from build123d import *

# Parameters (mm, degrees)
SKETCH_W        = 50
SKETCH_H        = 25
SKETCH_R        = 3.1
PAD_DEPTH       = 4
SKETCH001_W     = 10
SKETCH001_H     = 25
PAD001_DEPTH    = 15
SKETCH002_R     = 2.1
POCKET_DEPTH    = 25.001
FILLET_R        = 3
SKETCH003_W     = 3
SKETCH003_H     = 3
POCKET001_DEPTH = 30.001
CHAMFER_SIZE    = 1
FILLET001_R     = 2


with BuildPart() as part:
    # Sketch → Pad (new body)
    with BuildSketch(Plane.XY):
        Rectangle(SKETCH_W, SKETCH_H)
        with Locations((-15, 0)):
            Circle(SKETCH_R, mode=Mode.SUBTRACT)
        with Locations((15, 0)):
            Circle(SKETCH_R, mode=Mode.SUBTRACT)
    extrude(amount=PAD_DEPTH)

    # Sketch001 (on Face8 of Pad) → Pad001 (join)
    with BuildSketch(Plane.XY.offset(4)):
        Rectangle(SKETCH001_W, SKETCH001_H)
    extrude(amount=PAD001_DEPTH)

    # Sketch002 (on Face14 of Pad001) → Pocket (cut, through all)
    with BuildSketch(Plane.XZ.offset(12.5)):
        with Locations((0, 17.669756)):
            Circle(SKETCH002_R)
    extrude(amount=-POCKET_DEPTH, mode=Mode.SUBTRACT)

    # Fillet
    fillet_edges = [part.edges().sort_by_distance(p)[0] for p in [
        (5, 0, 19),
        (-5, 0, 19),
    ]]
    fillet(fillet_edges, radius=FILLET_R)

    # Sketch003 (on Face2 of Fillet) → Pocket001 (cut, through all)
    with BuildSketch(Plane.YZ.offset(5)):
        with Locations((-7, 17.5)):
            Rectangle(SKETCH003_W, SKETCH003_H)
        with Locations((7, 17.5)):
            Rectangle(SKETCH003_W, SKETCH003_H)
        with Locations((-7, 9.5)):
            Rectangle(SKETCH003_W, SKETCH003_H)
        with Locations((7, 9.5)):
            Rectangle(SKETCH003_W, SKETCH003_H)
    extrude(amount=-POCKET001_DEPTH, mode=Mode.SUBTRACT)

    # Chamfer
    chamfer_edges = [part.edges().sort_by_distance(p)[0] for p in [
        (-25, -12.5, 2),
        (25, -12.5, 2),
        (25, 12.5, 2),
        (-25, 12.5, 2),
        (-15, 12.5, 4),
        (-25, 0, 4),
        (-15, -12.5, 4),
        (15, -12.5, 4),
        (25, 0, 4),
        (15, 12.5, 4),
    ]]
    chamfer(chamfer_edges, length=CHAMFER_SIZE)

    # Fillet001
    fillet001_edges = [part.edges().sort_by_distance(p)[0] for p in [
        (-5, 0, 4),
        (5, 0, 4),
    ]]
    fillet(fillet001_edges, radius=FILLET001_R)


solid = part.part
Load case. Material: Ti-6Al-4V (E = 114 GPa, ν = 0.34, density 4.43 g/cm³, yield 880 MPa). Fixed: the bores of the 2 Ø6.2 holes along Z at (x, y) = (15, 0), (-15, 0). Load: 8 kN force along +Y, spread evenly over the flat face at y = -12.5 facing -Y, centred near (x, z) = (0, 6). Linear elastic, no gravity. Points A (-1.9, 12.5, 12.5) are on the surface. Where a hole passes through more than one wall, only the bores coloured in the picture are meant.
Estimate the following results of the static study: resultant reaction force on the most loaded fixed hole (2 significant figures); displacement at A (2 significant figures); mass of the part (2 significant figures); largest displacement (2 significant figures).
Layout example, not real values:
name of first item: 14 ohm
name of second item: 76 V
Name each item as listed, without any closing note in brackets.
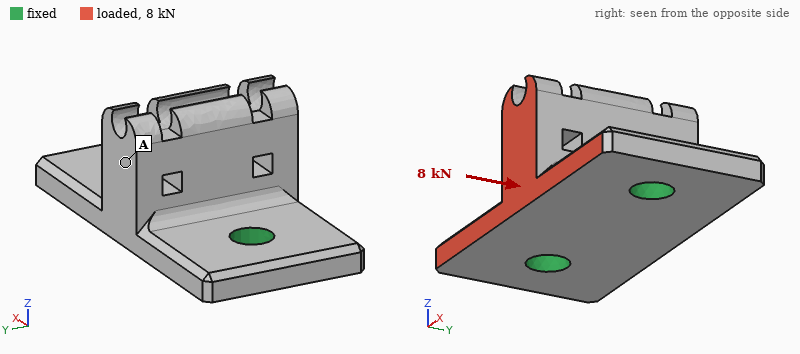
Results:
resultant reaction force on the most loaded fixed hole: 4.0 kN
displacement at A: 0.082 mm
mass of the part: 35 g
largest displacement: 0.11 mm
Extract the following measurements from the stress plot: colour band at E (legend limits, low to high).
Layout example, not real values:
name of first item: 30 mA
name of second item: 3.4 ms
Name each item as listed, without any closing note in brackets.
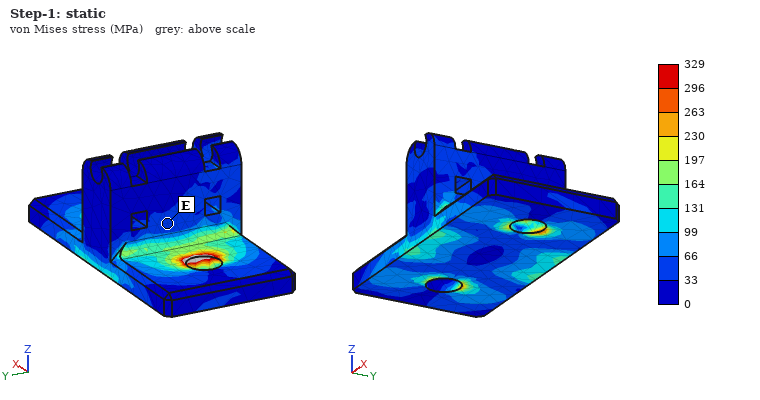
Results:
colour band at E: 33 to 66 MPa
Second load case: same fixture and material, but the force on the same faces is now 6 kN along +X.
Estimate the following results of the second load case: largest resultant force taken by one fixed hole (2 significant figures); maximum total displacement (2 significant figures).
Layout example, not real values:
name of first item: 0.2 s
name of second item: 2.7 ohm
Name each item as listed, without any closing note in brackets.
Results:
largest resultant force taken by one fixed hole: 3.9 kN
maximum total displacement: 55 µm
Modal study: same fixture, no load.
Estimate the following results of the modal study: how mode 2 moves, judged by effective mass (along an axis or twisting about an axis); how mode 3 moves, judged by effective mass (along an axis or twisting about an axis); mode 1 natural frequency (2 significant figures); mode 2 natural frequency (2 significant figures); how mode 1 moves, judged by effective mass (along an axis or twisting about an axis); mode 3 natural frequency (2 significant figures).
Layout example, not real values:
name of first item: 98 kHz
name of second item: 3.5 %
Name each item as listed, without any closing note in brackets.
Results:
how mode 2 moves, judged by effective mass: along Z
how mode 3 moves, judged by effective mass: along X
mode 1 natural frequency: 8400 Hz
mode 2 natural frequency: 16 kHz
how mode 1 moves, judged by effective mass: along Y
mode 3 natural frequency: 17 kHz
